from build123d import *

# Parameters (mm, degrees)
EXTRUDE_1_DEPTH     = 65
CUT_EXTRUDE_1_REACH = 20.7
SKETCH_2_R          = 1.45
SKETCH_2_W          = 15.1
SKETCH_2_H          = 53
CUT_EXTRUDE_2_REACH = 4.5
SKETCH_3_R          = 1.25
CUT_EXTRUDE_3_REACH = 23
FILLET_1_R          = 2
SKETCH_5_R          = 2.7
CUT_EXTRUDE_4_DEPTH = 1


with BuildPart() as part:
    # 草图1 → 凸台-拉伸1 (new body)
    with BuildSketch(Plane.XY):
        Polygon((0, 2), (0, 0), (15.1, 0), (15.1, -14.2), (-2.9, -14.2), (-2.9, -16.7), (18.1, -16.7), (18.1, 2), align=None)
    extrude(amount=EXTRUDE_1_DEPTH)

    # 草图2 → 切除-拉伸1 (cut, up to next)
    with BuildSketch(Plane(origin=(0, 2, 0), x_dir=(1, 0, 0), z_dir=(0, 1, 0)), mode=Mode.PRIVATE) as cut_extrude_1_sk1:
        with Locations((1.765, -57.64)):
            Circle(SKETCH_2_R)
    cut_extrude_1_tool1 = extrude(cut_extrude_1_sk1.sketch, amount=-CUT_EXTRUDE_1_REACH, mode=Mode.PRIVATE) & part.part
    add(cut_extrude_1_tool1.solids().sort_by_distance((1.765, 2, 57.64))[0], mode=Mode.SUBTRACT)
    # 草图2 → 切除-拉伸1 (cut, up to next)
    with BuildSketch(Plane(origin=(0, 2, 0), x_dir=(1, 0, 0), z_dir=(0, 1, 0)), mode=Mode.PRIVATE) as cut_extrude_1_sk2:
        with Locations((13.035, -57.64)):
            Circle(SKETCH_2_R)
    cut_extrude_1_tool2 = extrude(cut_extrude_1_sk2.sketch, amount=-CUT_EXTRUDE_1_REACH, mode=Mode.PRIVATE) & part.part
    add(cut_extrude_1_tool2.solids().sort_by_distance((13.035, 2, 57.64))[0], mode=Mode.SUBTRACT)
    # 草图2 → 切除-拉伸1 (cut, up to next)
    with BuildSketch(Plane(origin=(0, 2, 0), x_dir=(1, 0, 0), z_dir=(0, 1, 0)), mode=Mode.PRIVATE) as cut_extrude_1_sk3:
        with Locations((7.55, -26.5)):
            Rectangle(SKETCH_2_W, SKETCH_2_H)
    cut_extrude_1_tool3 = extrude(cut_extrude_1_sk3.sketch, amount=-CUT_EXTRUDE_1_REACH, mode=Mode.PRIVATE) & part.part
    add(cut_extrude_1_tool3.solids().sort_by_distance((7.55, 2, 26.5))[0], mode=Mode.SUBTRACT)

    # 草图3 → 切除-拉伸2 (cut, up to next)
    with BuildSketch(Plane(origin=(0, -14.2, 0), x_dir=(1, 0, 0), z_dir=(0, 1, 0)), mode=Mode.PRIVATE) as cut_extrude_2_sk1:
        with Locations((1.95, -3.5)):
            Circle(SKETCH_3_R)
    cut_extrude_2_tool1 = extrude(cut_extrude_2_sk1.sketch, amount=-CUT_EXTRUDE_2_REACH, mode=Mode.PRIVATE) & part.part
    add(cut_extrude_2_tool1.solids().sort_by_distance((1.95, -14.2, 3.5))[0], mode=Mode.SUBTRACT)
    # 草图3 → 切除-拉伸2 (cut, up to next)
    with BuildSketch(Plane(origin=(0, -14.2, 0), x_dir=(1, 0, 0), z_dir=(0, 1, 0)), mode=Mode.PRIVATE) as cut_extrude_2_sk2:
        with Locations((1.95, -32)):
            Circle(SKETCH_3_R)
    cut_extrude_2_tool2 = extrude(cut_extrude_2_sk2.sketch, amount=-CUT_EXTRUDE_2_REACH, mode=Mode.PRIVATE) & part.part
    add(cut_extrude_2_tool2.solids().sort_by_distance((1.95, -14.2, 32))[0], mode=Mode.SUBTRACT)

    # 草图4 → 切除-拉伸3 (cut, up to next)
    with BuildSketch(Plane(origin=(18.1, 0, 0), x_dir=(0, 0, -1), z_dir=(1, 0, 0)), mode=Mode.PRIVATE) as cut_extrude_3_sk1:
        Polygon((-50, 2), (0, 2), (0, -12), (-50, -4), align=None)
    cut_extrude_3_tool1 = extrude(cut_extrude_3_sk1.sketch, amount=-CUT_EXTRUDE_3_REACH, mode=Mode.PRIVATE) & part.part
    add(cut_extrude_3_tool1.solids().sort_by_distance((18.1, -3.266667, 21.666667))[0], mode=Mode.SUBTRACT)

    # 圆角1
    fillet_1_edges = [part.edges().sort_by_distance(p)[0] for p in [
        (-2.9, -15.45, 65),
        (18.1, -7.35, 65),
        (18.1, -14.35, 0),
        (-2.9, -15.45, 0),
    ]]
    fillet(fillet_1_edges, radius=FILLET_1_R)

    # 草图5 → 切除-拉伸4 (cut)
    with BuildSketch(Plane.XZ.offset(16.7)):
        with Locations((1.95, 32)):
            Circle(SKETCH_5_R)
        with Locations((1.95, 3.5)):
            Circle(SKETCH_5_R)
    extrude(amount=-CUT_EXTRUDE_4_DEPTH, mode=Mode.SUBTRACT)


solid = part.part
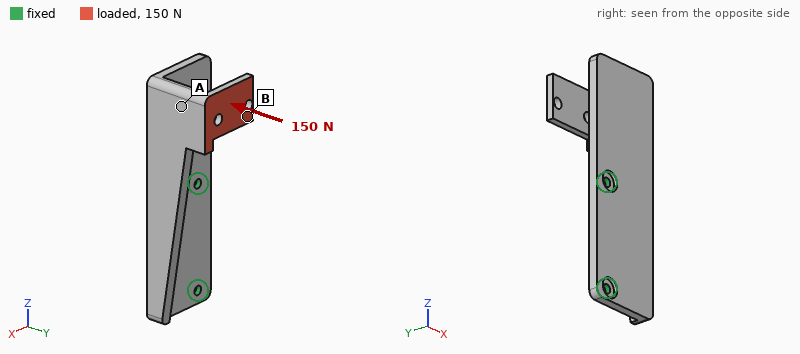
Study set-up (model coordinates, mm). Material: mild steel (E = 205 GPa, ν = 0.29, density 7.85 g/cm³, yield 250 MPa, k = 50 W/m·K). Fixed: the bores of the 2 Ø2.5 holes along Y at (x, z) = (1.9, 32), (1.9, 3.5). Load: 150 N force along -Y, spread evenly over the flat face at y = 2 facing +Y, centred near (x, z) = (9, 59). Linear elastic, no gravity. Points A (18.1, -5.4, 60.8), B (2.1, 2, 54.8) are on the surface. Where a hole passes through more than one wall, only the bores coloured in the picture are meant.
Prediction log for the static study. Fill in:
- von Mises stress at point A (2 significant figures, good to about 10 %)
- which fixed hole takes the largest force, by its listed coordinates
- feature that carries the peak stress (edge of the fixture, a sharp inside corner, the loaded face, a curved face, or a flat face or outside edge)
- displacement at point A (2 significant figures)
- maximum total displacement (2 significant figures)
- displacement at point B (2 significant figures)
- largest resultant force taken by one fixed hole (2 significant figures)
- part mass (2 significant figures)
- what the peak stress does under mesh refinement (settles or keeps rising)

40 MPa
(1.9, 32)
edge of the fixture
0.11 mm
0.18 mm
0.14 mm
290 N
42 g
keeps rising
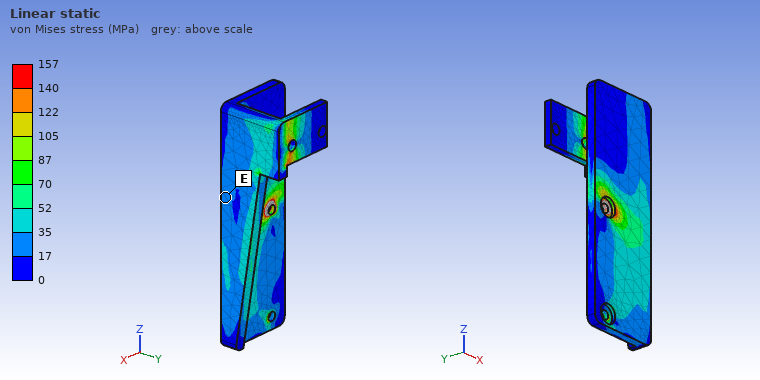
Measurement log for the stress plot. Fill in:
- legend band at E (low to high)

17 to 35 MPa
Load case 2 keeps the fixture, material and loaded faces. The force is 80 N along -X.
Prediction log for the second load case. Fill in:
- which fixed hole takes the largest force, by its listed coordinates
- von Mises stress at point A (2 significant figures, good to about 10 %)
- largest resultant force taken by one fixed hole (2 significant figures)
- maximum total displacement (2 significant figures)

(1.9, 32)
25 MPa
160 N
0.11 mm
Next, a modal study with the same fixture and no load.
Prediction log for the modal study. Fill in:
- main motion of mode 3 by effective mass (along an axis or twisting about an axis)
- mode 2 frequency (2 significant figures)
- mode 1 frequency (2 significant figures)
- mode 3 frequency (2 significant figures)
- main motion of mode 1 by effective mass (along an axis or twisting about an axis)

along Y
2200 Hz
1400 Hz
3800 Hz
along Y
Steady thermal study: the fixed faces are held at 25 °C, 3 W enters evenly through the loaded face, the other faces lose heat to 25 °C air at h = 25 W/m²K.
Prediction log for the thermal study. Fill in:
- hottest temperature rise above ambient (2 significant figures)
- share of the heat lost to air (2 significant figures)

48 K
43 %
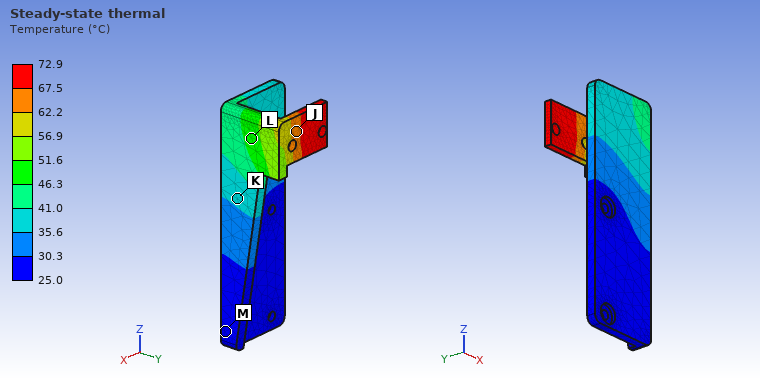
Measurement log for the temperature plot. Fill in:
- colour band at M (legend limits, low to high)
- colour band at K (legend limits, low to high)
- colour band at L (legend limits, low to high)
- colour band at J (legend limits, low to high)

25.0 to 30.3 °C
35.6 to 41.0 °C
46.3 to 51.6 °C
62.2 to 67.5 °C
